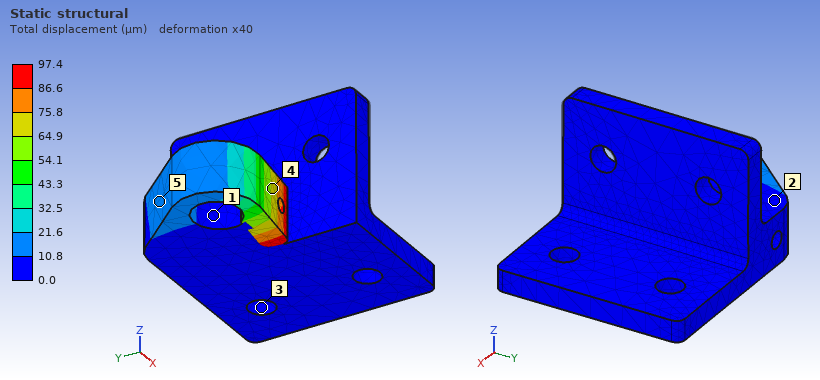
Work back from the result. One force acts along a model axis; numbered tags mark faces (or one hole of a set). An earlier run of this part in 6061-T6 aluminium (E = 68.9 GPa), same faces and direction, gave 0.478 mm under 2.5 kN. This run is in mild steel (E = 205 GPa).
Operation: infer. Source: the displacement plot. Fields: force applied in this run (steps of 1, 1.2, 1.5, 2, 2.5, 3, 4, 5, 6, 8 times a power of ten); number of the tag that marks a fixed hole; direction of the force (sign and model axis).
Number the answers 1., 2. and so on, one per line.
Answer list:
1. 1.5 kN
2. 3
3. +Y
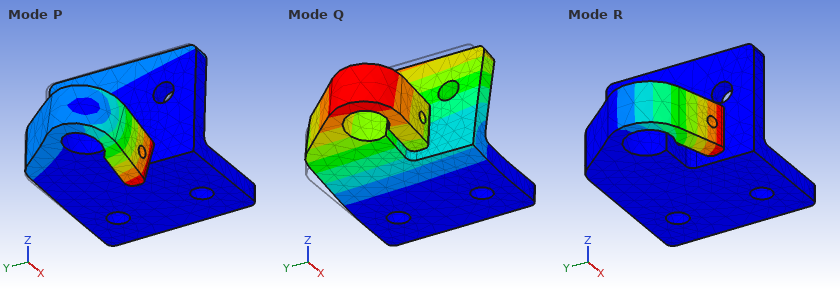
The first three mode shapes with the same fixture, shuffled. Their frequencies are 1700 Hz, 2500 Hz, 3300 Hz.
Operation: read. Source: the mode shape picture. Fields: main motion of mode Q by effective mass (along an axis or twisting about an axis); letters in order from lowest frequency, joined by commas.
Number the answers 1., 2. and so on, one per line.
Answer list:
1. along Z
2. Q, R, P
